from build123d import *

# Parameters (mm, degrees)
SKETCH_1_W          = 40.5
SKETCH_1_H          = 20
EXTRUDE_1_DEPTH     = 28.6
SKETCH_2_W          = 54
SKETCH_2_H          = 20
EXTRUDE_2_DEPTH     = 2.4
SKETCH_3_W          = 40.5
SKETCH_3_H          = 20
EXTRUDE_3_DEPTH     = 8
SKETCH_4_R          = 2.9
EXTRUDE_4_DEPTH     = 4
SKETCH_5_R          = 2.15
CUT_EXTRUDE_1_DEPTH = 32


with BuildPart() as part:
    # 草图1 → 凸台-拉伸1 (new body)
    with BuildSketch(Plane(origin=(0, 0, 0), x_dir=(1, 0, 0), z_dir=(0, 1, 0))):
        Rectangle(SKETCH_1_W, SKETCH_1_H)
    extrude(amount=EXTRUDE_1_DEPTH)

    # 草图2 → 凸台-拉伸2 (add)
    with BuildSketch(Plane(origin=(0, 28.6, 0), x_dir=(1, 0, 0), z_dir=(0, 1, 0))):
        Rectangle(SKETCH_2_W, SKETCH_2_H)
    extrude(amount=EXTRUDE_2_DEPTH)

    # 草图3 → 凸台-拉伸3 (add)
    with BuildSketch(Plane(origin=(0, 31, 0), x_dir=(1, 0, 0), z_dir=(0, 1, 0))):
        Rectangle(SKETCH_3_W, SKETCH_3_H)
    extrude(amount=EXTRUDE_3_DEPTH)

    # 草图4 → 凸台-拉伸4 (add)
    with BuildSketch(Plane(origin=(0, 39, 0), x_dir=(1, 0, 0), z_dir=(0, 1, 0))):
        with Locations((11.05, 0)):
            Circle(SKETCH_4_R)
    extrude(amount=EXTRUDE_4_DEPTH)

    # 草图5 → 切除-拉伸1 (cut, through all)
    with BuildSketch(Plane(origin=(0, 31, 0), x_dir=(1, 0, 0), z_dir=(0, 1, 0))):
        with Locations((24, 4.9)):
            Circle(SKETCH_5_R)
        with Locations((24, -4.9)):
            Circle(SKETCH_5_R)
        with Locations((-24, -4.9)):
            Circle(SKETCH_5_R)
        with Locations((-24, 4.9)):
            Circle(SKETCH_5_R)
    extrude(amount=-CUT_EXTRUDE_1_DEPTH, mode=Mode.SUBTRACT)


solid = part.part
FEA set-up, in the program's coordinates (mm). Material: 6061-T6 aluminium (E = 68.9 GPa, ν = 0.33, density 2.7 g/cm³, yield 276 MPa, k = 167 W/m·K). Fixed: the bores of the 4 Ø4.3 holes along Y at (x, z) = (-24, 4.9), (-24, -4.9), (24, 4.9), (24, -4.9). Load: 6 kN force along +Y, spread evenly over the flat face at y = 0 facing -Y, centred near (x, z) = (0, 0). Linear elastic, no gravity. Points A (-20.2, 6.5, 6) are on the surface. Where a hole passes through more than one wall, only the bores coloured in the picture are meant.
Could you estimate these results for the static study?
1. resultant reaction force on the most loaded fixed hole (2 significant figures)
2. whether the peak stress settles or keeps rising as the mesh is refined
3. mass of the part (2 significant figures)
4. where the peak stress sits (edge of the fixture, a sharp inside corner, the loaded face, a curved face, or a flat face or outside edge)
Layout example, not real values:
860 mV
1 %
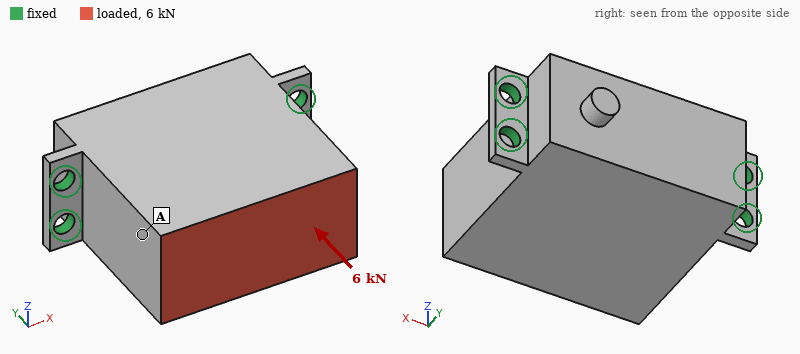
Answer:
1.5 kN
keeps rising
87 g
edge of the fixture
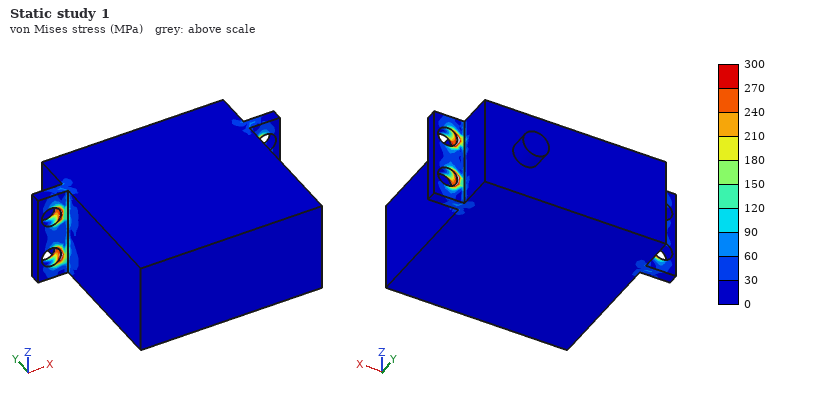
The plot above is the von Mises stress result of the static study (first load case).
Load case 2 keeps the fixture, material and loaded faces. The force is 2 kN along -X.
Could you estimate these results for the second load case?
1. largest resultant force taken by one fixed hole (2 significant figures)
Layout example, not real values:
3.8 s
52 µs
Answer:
870 N
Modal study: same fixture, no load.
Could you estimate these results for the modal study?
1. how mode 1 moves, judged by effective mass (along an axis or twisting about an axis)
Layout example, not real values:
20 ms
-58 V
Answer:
along Z
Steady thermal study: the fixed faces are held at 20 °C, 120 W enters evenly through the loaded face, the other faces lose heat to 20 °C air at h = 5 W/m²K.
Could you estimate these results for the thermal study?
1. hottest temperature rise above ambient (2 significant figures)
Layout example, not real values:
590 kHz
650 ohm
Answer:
60 K
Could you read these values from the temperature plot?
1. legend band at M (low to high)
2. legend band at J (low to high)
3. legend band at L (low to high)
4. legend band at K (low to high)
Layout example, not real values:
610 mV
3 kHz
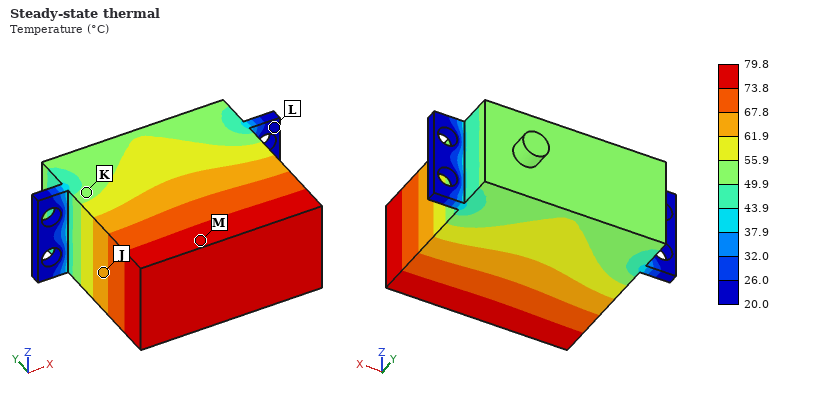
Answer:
73.8 to 79.8 °C
61.9 to 67.8 °C
20.0 to 26.0 °C
49.9 to 55.9 °C
